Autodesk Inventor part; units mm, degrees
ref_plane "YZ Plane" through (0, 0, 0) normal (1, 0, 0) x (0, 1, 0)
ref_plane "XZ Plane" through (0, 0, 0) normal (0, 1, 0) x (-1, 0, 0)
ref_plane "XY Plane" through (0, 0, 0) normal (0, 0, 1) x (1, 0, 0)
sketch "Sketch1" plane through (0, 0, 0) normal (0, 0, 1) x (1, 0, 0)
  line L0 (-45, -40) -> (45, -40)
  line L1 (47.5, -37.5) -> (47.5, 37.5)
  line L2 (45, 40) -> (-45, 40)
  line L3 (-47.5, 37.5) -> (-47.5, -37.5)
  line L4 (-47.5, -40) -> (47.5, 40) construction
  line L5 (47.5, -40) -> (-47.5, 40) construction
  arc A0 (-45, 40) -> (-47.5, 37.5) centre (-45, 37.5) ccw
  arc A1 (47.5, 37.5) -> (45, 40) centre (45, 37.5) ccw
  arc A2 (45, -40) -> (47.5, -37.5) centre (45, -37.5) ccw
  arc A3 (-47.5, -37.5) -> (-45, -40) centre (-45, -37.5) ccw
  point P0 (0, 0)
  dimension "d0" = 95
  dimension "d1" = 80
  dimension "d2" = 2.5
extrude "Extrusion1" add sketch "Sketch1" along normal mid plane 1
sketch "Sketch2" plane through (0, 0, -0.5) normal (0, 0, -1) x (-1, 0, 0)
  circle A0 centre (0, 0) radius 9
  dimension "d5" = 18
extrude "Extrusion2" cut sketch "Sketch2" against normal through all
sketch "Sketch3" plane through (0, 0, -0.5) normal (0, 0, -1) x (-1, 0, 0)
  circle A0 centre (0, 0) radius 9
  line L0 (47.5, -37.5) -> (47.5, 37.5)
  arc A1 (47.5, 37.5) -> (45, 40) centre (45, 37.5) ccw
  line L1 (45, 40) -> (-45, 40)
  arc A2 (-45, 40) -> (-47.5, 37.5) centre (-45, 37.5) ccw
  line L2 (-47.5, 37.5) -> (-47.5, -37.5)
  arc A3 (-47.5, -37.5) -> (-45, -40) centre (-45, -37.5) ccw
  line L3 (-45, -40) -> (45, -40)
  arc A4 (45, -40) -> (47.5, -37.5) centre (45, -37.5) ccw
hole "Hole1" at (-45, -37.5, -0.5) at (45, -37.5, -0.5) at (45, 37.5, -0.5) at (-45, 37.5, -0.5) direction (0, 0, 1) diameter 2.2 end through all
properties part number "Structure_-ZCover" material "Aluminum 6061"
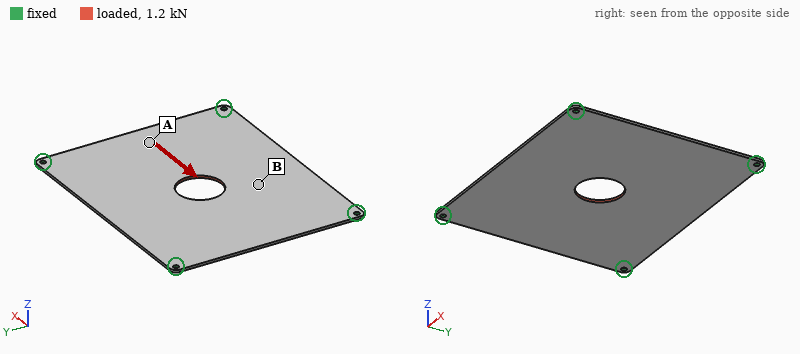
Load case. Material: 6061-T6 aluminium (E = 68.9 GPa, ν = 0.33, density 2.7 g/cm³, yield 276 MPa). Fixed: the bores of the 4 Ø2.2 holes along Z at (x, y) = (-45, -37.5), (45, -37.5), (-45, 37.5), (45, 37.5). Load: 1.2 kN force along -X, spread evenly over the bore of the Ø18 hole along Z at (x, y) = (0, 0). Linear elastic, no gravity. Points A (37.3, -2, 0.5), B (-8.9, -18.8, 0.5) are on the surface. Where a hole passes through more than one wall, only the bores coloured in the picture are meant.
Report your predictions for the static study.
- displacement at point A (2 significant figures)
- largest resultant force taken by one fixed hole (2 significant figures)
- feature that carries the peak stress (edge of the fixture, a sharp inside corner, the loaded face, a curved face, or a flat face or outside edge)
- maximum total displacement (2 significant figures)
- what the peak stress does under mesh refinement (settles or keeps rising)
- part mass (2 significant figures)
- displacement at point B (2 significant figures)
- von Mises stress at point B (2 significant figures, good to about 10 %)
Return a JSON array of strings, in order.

["14 µm", "340 N", "edge of the fixture", "18 µm", "keeps rising", "20 g", "13 µm", "13 MPa"]
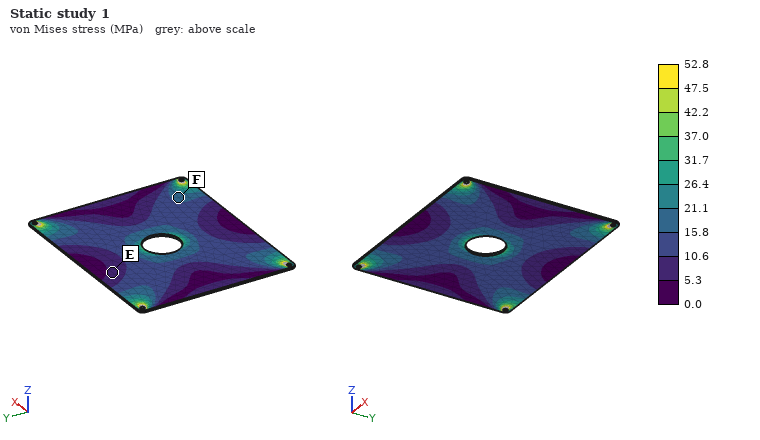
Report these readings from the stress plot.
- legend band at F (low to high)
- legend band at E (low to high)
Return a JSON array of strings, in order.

["15.8 to 21.1 MPa", "5.3 to 10.6 MPa"]
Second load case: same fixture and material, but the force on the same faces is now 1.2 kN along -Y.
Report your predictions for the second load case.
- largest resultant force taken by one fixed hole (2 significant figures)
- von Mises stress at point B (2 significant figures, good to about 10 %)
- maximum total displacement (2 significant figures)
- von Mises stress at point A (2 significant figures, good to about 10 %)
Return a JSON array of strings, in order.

["360 N", "14 MPa", "23 µm", "9.3 MPa"]
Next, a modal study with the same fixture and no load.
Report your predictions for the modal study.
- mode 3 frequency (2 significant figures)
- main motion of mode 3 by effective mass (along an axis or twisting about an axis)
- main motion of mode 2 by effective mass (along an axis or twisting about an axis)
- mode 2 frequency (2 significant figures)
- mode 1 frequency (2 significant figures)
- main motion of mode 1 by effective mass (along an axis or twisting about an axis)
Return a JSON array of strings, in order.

["890 Hz", "twisting about Y", "twisting about X", "750 Hz", "420 Hz", "along Z"]
